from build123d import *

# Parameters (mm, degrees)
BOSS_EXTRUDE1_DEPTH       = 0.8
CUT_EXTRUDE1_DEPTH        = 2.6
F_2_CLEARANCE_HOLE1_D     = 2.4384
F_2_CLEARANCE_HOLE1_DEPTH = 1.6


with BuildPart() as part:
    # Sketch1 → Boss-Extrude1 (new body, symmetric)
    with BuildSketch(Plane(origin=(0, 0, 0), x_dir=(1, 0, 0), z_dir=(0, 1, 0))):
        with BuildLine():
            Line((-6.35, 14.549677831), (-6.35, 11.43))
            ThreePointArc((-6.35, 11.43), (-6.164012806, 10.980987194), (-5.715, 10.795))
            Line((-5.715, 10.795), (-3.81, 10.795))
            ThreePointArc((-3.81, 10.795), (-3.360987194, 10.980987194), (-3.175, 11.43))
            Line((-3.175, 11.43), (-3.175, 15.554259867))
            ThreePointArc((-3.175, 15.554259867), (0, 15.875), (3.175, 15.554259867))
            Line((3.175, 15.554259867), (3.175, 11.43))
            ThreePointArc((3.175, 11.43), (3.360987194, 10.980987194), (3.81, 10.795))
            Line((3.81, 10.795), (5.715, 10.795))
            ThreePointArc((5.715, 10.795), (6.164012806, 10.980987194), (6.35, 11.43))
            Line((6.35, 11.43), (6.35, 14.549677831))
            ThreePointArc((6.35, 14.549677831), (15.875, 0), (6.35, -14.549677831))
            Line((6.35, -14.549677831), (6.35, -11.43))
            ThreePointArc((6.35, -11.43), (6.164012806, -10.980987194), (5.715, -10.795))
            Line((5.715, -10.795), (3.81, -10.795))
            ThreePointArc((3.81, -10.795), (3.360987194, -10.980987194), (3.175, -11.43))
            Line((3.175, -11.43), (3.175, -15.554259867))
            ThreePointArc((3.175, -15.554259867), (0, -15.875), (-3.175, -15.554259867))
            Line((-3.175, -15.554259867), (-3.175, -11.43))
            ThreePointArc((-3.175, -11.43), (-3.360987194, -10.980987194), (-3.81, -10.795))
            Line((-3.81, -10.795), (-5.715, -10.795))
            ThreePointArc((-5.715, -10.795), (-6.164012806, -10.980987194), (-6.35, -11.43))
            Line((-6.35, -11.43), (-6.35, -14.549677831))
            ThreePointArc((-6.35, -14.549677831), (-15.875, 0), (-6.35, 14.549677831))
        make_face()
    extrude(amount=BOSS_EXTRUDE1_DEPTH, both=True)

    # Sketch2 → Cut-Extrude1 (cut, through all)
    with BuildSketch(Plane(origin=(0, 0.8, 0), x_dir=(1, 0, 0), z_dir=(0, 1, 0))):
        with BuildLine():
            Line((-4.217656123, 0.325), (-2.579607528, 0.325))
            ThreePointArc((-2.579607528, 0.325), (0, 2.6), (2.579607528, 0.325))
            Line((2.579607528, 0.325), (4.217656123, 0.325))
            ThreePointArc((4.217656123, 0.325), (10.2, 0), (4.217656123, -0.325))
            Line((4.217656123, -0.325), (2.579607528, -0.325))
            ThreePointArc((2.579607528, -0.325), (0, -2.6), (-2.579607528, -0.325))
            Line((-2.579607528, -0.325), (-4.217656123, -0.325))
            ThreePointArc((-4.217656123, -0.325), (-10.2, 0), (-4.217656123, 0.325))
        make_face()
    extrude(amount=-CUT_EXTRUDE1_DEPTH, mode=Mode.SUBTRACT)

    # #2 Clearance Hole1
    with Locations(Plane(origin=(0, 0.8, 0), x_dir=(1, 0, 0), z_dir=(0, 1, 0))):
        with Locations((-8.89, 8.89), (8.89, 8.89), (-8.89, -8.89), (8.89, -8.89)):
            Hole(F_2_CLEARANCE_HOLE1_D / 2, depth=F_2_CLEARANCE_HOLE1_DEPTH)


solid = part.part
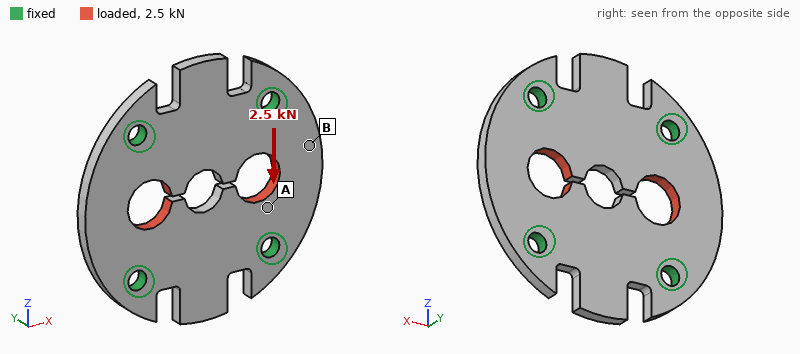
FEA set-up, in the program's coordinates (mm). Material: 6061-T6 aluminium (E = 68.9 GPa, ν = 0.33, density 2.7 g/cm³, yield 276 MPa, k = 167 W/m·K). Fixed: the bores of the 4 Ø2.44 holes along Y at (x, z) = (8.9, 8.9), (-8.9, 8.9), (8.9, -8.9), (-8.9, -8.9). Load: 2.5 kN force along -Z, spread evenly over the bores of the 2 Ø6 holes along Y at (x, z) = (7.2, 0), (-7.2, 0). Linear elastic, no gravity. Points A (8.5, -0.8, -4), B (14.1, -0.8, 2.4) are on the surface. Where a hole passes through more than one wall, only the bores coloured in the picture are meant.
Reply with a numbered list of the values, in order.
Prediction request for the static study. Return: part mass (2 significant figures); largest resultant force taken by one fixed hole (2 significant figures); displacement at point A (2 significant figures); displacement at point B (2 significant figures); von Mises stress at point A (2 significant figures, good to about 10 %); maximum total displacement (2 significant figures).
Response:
1. 2.8 g
2. 640 N
3. 3.6 µm
4. 2.6 µm
5. 54 MPa
6. 8.2 µm
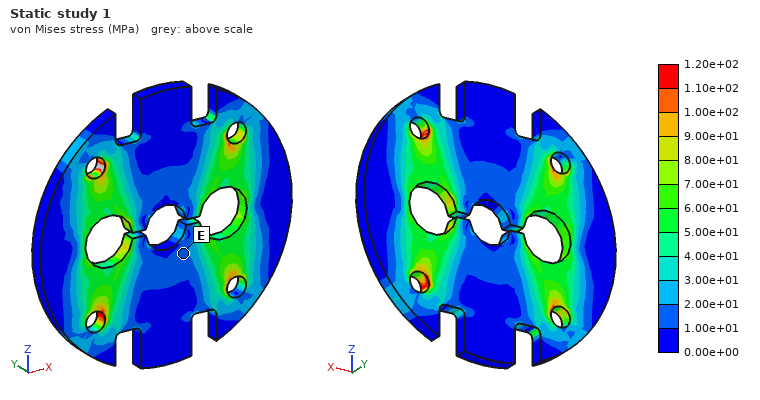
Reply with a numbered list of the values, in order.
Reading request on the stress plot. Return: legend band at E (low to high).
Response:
1. 1.00e+01 to 2.00e+01 MPa
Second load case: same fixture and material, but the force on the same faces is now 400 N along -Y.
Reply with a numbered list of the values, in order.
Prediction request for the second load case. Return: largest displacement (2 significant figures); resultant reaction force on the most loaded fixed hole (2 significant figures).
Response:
1. 58 µm
2. 100 N
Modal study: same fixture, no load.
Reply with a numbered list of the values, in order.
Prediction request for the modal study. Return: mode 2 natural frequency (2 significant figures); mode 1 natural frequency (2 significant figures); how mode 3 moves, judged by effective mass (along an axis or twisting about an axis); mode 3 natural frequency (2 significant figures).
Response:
1. 16 kHz
2. 16 kHz
3. along Y
4. 19 kHz
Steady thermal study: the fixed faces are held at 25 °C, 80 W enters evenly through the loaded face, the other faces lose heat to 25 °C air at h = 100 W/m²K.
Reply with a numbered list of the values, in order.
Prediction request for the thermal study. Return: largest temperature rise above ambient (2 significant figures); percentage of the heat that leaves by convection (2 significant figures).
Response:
1. 55 K
2. 4.3 %
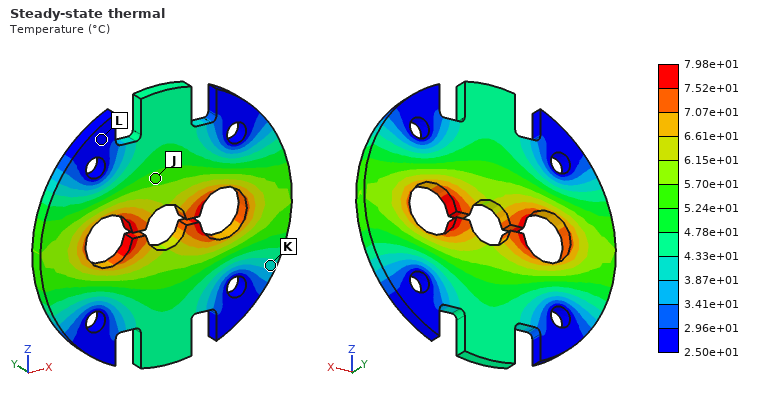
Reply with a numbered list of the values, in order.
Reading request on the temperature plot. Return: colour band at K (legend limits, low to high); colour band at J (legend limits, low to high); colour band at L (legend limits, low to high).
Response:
1. 3.87e+01 to 4.33e+01 °C
2. 5.24e+01 to 5.70e+01 °C
3. 2.50e+01 to 2.96e+01 °C
